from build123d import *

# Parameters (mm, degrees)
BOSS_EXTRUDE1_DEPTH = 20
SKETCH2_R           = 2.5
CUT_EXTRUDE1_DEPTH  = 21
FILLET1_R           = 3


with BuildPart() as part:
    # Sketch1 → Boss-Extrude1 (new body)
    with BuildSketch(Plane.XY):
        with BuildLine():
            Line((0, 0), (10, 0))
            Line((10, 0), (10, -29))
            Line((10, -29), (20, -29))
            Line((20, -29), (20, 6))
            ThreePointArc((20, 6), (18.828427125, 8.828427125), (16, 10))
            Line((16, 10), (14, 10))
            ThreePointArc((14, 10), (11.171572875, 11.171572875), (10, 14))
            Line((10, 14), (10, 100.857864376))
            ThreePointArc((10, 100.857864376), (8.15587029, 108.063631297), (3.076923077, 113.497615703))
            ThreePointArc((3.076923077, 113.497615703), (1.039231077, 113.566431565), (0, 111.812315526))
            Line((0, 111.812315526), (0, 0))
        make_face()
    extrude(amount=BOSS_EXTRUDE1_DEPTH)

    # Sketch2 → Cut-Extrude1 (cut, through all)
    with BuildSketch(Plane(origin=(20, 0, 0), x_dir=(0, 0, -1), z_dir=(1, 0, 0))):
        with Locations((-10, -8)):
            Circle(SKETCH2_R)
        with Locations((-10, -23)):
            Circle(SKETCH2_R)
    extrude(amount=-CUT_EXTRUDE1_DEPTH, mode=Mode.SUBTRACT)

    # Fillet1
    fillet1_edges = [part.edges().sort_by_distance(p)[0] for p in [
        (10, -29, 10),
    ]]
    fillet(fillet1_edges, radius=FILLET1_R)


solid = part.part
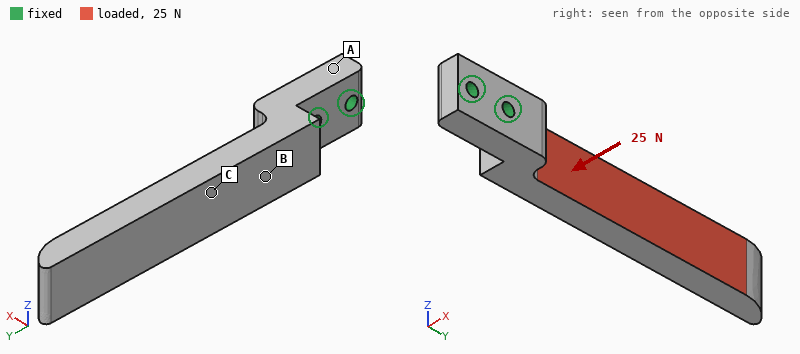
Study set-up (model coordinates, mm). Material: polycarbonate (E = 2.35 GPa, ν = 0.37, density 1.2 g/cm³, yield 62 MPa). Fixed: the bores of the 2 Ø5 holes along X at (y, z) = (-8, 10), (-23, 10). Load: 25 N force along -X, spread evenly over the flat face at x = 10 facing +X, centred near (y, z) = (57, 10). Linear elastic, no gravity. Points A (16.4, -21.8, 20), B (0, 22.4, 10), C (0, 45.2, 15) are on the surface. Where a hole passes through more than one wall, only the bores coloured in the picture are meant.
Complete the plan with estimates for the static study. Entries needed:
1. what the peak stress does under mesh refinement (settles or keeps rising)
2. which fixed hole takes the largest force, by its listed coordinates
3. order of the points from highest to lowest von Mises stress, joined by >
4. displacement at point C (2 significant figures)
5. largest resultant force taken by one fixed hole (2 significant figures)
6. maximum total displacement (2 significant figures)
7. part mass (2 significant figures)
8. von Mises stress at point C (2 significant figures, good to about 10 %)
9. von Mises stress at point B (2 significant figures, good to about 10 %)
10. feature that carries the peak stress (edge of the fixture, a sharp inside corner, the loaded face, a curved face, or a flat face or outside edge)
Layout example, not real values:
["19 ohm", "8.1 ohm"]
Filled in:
["keeps rising", "(-8, 10)", "B > C > A", "0.46 mm", "51 N", "1.5 mm", "35 g", "1.3 MPa", "2.6 MPa", "edge of the fixture"]
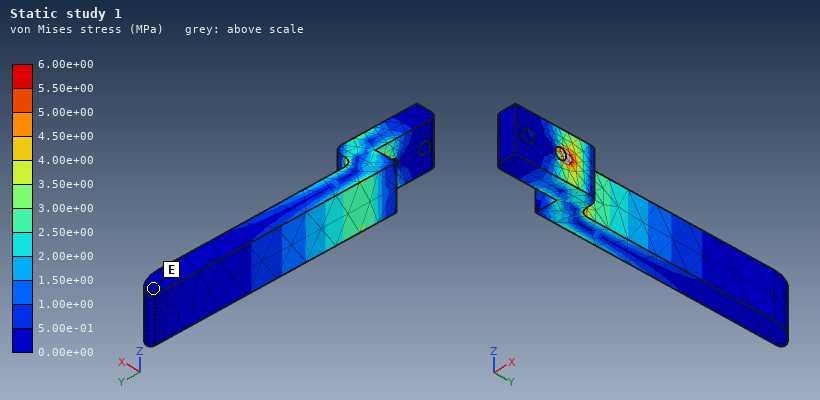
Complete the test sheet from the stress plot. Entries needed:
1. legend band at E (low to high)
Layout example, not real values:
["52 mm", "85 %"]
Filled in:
["0.00e+00 to 5.00e-01 MPa"]
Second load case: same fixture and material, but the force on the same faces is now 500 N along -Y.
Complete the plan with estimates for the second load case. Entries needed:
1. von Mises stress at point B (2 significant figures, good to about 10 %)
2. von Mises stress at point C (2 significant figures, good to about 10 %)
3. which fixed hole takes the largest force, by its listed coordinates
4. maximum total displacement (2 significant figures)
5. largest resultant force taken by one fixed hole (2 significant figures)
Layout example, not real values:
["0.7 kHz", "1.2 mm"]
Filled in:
["4.4 MPa", "3.2 MPa", "(-8, 10)", "1.4 mm", "420 N"]
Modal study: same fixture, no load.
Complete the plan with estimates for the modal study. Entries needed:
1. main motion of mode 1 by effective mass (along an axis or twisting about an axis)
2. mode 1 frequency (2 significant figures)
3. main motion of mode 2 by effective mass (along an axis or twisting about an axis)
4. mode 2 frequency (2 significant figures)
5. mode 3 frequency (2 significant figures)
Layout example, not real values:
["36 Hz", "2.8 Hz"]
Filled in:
["along X", "160 Hz", "along Z", "260 Hz", "910 Hz"]
